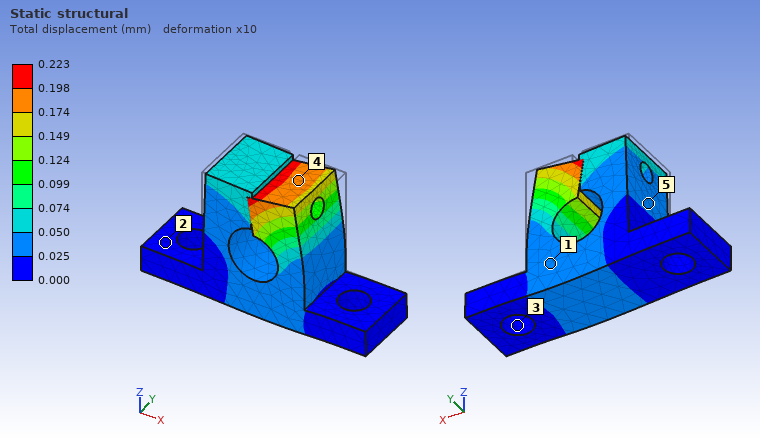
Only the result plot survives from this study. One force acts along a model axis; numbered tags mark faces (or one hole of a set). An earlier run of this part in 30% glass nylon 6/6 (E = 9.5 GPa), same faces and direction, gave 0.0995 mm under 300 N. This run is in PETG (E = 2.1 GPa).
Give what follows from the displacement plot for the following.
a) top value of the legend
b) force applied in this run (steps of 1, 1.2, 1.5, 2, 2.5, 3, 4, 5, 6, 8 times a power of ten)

0.223 mm
150 N
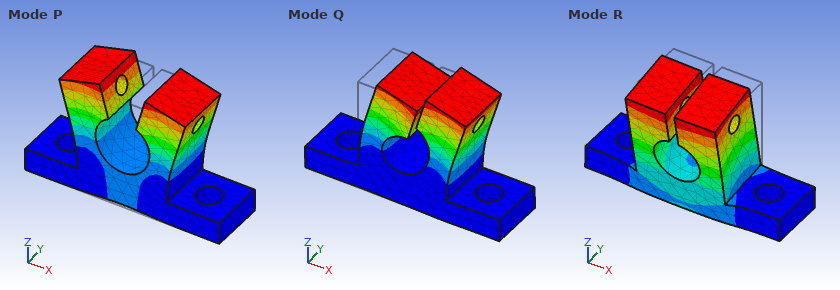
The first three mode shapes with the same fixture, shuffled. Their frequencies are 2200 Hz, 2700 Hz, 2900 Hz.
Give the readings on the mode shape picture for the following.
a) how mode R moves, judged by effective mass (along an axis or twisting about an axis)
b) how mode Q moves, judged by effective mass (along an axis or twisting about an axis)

along Y
along X
